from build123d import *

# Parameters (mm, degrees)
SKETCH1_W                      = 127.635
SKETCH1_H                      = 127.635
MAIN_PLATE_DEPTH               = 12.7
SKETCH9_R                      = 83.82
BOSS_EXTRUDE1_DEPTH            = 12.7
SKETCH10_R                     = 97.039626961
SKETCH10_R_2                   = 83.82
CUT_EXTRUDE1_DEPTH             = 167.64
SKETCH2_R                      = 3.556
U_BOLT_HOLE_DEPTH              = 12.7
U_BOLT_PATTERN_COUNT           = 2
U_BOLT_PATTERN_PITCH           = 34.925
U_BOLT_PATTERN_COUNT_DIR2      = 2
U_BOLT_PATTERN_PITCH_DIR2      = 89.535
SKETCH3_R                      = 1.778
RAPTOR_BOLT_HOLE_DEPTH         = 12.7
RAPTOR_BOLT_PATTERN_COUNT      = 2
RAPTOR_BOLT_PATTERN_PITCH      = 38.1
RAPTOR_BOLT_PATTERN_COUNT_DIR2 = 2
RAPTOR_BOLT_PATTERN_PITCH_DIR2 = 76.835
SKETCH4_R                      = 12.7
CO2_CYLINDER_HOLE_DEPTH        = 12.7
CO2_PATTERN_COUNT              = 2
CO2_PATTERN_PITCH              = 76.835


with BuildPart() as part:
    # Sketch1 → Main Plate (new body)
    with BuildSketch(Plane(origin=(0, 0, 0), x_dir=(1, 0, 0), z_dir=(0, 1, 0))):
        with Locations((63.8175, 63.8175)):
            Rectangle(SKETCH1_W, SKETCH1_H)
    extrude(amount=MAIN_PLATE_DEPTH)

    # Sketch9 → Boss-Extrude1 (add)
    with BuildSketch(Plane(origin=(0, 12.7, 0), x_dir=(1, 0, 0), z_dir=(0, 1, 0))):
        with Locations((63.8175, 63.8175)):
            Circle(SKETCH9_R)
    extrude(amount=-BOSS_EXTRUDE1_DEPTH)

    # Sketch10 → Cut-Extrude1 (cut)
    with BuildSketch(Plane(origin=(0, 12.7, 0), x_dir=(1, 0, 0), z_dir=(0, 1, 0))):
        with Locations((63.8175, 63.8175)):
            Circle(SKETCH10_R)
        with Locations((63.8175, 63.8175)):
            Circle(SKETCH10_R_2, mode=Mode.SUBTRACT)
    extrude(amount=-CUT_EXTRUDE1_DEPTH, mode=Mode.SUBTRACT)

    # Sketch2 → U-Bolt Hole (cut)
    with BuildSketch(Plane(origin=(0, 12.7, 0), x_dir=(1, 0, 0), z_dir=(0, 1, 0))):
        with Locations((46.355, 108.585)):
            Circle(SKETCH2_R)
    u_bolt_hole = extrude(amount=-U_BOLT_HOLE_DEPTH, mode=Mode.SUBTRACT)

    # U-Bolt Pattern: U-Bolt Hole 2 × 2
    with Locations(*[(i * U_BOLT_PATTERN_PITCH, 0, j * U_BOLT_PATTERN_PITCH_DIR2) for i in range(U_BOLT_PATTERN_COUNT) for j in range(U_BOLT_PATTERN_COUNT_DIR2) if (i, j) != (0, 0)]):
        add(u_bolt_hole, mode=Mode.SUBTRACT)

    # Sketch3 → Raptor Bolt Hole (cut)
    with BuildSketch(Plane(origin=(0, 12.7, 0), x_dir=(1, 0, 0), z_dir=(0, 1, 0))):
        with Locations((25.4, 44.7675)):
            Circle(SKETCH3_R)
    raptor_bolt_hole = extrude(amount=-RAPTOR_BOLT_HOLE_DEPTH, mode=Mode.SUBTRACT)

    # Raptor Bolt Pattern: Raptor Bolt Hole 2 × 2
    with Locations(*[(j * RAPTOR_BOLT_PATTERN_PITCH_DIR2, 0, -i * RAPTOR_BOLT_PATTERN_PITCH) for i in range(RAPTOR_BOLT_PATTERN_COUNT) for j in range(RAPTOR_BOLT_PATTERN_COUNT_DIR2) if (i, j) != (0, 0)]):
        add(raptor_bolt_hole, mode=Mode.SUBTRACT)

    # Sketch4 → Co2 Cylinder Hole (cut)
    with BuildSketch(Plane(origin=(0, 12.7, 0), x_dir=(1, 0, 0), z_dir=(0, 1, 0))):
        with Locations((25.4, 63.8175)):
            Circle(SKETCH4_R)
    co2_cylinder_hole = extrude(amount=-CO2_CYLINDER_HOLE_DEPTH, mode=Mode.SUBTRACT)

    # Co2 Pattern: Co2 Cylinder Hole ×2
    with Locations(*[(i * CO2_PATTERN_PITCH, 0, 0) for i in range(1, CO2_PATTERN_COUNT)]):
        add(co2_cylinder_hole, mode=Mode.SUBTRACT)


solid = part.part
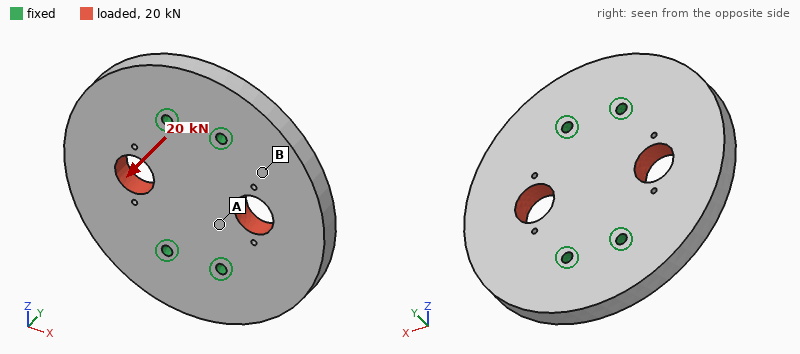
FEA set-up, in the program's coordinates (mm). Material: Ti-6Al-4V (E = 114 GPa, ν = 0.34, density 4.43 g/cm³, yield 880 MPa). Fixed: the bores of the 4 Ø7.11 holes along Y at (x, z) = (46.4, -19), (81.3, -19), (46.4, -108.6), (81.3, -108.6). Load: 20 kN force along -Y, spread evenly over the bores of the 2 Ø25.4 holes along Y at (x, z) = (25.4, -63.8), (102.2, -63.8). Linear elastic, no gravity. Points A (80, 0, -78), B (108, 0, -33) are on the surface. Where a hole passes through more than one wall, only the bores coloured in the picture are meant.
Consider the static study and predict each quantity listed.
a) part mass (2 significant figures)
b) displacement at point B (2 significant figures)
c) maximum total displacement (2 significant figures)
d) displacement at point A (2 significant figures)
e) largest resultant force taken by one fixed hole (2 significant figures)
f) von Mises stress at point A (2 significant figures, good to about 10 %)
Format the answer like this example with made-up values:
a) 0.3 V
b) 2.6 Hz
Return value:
a) 1.2 kg
b) 0.051 mm
c) 0.13 mm
d) 0.038 mm
e) 5.0 kN
f) 51 MPa
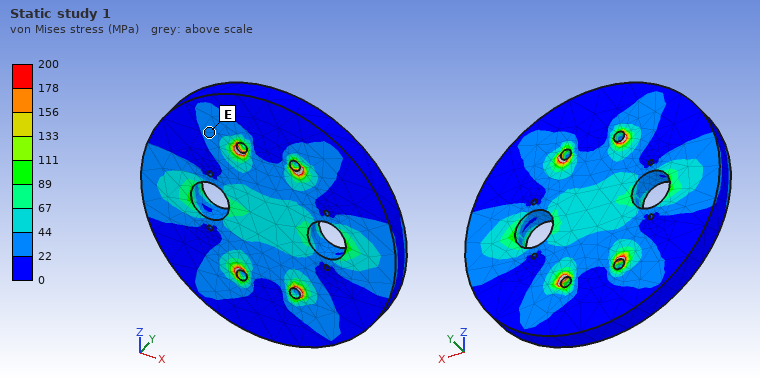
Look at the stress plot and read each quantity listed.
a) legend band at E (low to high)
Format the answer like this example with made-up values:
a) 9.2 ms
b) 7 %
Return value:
a) 22 to 44 MPa
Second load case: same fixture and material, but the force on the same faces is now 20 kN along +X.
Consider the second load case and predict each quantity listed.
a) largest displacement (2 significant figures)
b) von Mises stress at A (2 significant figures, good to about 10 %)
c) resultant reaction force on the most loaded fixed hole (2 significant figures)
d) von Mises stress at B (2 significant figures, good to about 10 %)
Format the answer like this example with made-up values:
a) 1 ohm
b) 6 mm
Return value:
a) 7.4 µm
b) 9.1 MPa
c) 5.0 kN
d) 8.9 MPa
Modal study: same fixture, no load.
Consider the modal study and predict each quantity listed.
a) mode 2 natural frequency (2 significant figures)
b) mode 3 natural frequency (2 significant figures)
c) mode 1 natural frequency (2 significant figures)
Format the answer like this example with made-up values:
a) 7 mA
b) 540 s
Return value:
a) 2400 Hz
b) 4800 Hz
c) 2400 Hz
